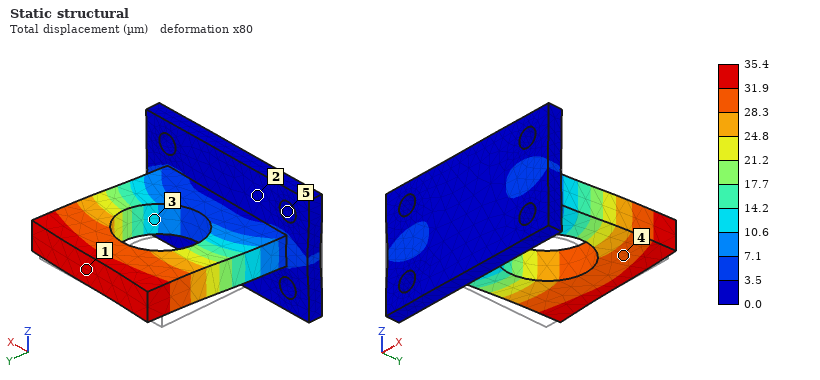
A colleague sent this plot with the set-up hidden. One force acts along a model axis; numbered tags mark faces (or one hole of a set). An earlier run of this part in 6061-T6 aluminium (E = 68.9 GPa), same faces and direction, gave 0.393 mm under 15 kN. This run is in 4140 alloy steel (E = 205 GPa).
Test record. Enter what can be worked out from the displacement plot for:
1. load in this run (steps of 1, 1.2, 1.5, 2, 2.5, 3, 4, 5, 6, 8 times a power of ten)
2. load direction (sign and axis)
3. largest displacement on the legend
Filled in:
4 kN
+X
35.4 µm
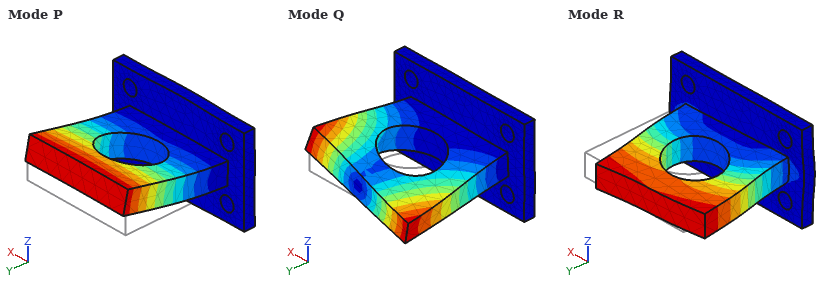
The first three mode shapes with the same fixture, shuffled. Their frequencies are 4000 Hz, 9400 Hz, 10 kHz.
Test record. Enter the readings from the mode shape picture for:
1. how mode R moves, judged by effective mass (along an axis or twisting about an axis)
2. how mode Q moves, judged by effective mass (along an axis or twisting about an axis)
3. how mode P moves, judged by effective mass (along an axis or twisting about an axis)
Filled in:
along X
twisting about Y
along Z
